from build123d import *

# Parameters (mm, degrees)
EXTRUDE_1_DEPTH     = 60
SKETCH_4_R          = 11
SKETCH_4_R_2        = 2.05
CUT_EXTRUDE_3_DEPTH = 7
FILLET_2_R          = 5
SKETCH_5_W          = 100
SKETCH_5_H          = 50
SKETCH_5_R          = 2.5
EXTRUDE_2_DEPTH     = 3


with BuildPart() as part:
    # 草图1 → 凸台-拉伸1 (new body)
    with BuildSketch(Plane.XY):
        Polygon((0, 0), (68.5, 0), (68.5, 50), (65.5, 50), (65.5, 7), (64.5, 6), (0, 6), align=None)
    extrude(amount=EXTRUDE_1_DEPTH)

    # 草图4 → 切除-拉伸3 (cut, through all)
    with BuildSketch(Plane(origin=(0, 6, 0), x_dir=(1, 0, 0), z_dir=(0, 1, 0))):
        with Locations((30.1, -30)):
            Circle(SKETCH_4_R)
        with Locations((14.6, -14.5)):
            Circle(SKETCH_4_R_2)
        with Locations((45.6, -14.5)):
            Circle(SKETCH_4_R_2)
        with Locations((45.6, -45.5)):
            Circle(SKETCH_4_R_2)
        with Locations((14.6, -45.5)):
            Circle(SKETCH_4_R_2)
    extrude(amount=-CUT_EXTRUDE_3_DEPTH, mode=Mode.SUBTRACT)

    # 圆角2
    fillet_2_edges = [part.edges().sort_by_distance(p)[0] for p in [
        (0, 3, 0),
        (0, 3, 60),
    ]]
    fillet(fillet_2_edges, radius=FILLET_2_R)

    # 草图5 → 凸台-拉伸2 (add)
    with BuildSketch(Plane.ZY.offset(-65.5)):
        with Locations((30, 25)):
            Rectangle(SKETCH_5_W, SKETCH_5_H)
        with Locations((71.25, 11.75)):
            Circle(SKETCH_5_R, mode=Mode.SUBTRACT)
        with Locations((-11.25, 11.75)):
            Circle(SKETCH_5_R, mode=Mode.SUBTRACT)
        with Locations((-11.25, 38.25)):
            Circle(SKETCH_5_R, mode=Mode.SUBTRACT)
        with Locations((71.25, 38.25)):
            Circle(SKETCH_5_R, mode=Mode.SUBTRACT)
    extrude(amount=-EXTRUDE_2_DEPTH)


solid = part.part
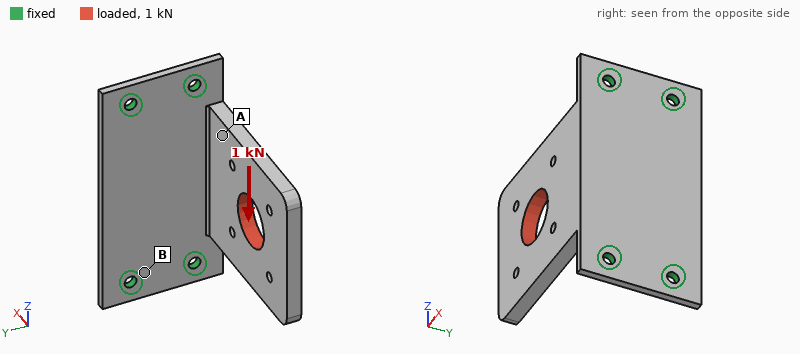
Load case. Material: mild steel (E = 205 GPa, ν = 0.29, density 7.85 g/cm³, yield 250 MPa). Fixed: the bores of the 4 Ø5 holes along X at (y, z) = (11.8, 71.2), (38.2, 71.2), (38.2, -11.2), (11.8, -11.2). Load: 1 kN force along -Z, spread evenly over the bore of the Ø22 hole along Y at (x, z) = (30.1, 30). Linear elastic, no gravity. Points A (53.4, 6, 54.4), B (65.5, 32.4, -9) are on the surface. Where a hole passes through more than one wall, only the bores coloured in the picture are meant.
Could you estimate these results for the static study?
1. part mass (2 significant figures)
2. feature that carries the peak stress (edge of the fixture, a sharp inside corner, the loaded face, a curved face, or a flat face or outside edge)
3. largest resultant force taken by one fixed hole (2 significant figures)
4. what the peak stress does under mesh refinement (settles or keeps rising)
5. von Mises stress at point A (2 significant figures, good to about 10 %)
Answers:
280 g
edge of the fixture
700 N
keeps rising
20 MPa
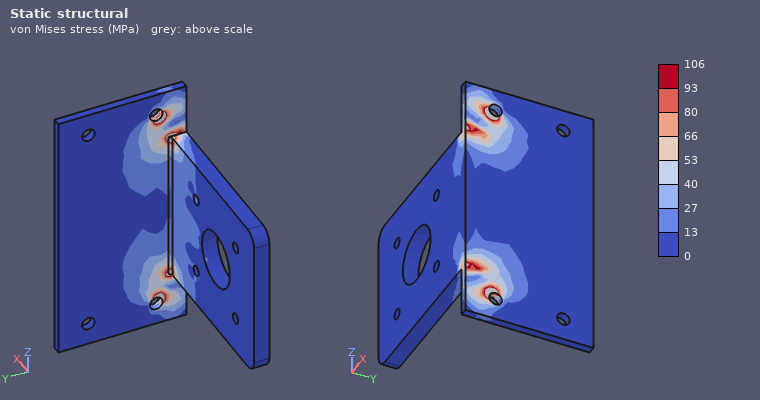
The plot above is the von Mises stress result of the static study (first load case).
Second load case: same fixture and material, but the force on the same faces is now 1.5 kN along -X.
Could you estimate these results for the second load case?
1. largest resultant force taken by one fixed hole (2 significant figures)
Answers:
950 N
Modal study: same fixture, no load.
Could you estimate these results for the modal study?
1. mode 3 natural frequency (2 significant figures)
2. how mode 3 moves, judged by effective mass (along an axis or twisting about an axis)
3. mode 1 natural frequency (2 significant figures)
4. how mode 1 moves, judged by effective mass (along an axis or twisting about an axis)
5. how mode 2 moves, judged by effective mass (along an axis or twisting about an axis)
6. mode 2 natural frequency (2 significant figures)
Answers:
2400 Hz
along X
500 Hz
along Y
along Z
1900 Hz
